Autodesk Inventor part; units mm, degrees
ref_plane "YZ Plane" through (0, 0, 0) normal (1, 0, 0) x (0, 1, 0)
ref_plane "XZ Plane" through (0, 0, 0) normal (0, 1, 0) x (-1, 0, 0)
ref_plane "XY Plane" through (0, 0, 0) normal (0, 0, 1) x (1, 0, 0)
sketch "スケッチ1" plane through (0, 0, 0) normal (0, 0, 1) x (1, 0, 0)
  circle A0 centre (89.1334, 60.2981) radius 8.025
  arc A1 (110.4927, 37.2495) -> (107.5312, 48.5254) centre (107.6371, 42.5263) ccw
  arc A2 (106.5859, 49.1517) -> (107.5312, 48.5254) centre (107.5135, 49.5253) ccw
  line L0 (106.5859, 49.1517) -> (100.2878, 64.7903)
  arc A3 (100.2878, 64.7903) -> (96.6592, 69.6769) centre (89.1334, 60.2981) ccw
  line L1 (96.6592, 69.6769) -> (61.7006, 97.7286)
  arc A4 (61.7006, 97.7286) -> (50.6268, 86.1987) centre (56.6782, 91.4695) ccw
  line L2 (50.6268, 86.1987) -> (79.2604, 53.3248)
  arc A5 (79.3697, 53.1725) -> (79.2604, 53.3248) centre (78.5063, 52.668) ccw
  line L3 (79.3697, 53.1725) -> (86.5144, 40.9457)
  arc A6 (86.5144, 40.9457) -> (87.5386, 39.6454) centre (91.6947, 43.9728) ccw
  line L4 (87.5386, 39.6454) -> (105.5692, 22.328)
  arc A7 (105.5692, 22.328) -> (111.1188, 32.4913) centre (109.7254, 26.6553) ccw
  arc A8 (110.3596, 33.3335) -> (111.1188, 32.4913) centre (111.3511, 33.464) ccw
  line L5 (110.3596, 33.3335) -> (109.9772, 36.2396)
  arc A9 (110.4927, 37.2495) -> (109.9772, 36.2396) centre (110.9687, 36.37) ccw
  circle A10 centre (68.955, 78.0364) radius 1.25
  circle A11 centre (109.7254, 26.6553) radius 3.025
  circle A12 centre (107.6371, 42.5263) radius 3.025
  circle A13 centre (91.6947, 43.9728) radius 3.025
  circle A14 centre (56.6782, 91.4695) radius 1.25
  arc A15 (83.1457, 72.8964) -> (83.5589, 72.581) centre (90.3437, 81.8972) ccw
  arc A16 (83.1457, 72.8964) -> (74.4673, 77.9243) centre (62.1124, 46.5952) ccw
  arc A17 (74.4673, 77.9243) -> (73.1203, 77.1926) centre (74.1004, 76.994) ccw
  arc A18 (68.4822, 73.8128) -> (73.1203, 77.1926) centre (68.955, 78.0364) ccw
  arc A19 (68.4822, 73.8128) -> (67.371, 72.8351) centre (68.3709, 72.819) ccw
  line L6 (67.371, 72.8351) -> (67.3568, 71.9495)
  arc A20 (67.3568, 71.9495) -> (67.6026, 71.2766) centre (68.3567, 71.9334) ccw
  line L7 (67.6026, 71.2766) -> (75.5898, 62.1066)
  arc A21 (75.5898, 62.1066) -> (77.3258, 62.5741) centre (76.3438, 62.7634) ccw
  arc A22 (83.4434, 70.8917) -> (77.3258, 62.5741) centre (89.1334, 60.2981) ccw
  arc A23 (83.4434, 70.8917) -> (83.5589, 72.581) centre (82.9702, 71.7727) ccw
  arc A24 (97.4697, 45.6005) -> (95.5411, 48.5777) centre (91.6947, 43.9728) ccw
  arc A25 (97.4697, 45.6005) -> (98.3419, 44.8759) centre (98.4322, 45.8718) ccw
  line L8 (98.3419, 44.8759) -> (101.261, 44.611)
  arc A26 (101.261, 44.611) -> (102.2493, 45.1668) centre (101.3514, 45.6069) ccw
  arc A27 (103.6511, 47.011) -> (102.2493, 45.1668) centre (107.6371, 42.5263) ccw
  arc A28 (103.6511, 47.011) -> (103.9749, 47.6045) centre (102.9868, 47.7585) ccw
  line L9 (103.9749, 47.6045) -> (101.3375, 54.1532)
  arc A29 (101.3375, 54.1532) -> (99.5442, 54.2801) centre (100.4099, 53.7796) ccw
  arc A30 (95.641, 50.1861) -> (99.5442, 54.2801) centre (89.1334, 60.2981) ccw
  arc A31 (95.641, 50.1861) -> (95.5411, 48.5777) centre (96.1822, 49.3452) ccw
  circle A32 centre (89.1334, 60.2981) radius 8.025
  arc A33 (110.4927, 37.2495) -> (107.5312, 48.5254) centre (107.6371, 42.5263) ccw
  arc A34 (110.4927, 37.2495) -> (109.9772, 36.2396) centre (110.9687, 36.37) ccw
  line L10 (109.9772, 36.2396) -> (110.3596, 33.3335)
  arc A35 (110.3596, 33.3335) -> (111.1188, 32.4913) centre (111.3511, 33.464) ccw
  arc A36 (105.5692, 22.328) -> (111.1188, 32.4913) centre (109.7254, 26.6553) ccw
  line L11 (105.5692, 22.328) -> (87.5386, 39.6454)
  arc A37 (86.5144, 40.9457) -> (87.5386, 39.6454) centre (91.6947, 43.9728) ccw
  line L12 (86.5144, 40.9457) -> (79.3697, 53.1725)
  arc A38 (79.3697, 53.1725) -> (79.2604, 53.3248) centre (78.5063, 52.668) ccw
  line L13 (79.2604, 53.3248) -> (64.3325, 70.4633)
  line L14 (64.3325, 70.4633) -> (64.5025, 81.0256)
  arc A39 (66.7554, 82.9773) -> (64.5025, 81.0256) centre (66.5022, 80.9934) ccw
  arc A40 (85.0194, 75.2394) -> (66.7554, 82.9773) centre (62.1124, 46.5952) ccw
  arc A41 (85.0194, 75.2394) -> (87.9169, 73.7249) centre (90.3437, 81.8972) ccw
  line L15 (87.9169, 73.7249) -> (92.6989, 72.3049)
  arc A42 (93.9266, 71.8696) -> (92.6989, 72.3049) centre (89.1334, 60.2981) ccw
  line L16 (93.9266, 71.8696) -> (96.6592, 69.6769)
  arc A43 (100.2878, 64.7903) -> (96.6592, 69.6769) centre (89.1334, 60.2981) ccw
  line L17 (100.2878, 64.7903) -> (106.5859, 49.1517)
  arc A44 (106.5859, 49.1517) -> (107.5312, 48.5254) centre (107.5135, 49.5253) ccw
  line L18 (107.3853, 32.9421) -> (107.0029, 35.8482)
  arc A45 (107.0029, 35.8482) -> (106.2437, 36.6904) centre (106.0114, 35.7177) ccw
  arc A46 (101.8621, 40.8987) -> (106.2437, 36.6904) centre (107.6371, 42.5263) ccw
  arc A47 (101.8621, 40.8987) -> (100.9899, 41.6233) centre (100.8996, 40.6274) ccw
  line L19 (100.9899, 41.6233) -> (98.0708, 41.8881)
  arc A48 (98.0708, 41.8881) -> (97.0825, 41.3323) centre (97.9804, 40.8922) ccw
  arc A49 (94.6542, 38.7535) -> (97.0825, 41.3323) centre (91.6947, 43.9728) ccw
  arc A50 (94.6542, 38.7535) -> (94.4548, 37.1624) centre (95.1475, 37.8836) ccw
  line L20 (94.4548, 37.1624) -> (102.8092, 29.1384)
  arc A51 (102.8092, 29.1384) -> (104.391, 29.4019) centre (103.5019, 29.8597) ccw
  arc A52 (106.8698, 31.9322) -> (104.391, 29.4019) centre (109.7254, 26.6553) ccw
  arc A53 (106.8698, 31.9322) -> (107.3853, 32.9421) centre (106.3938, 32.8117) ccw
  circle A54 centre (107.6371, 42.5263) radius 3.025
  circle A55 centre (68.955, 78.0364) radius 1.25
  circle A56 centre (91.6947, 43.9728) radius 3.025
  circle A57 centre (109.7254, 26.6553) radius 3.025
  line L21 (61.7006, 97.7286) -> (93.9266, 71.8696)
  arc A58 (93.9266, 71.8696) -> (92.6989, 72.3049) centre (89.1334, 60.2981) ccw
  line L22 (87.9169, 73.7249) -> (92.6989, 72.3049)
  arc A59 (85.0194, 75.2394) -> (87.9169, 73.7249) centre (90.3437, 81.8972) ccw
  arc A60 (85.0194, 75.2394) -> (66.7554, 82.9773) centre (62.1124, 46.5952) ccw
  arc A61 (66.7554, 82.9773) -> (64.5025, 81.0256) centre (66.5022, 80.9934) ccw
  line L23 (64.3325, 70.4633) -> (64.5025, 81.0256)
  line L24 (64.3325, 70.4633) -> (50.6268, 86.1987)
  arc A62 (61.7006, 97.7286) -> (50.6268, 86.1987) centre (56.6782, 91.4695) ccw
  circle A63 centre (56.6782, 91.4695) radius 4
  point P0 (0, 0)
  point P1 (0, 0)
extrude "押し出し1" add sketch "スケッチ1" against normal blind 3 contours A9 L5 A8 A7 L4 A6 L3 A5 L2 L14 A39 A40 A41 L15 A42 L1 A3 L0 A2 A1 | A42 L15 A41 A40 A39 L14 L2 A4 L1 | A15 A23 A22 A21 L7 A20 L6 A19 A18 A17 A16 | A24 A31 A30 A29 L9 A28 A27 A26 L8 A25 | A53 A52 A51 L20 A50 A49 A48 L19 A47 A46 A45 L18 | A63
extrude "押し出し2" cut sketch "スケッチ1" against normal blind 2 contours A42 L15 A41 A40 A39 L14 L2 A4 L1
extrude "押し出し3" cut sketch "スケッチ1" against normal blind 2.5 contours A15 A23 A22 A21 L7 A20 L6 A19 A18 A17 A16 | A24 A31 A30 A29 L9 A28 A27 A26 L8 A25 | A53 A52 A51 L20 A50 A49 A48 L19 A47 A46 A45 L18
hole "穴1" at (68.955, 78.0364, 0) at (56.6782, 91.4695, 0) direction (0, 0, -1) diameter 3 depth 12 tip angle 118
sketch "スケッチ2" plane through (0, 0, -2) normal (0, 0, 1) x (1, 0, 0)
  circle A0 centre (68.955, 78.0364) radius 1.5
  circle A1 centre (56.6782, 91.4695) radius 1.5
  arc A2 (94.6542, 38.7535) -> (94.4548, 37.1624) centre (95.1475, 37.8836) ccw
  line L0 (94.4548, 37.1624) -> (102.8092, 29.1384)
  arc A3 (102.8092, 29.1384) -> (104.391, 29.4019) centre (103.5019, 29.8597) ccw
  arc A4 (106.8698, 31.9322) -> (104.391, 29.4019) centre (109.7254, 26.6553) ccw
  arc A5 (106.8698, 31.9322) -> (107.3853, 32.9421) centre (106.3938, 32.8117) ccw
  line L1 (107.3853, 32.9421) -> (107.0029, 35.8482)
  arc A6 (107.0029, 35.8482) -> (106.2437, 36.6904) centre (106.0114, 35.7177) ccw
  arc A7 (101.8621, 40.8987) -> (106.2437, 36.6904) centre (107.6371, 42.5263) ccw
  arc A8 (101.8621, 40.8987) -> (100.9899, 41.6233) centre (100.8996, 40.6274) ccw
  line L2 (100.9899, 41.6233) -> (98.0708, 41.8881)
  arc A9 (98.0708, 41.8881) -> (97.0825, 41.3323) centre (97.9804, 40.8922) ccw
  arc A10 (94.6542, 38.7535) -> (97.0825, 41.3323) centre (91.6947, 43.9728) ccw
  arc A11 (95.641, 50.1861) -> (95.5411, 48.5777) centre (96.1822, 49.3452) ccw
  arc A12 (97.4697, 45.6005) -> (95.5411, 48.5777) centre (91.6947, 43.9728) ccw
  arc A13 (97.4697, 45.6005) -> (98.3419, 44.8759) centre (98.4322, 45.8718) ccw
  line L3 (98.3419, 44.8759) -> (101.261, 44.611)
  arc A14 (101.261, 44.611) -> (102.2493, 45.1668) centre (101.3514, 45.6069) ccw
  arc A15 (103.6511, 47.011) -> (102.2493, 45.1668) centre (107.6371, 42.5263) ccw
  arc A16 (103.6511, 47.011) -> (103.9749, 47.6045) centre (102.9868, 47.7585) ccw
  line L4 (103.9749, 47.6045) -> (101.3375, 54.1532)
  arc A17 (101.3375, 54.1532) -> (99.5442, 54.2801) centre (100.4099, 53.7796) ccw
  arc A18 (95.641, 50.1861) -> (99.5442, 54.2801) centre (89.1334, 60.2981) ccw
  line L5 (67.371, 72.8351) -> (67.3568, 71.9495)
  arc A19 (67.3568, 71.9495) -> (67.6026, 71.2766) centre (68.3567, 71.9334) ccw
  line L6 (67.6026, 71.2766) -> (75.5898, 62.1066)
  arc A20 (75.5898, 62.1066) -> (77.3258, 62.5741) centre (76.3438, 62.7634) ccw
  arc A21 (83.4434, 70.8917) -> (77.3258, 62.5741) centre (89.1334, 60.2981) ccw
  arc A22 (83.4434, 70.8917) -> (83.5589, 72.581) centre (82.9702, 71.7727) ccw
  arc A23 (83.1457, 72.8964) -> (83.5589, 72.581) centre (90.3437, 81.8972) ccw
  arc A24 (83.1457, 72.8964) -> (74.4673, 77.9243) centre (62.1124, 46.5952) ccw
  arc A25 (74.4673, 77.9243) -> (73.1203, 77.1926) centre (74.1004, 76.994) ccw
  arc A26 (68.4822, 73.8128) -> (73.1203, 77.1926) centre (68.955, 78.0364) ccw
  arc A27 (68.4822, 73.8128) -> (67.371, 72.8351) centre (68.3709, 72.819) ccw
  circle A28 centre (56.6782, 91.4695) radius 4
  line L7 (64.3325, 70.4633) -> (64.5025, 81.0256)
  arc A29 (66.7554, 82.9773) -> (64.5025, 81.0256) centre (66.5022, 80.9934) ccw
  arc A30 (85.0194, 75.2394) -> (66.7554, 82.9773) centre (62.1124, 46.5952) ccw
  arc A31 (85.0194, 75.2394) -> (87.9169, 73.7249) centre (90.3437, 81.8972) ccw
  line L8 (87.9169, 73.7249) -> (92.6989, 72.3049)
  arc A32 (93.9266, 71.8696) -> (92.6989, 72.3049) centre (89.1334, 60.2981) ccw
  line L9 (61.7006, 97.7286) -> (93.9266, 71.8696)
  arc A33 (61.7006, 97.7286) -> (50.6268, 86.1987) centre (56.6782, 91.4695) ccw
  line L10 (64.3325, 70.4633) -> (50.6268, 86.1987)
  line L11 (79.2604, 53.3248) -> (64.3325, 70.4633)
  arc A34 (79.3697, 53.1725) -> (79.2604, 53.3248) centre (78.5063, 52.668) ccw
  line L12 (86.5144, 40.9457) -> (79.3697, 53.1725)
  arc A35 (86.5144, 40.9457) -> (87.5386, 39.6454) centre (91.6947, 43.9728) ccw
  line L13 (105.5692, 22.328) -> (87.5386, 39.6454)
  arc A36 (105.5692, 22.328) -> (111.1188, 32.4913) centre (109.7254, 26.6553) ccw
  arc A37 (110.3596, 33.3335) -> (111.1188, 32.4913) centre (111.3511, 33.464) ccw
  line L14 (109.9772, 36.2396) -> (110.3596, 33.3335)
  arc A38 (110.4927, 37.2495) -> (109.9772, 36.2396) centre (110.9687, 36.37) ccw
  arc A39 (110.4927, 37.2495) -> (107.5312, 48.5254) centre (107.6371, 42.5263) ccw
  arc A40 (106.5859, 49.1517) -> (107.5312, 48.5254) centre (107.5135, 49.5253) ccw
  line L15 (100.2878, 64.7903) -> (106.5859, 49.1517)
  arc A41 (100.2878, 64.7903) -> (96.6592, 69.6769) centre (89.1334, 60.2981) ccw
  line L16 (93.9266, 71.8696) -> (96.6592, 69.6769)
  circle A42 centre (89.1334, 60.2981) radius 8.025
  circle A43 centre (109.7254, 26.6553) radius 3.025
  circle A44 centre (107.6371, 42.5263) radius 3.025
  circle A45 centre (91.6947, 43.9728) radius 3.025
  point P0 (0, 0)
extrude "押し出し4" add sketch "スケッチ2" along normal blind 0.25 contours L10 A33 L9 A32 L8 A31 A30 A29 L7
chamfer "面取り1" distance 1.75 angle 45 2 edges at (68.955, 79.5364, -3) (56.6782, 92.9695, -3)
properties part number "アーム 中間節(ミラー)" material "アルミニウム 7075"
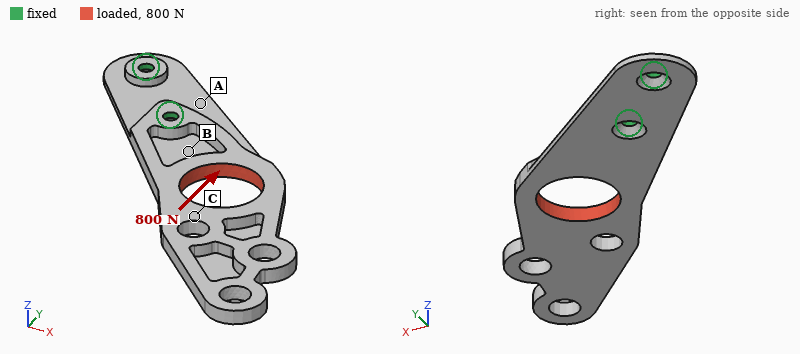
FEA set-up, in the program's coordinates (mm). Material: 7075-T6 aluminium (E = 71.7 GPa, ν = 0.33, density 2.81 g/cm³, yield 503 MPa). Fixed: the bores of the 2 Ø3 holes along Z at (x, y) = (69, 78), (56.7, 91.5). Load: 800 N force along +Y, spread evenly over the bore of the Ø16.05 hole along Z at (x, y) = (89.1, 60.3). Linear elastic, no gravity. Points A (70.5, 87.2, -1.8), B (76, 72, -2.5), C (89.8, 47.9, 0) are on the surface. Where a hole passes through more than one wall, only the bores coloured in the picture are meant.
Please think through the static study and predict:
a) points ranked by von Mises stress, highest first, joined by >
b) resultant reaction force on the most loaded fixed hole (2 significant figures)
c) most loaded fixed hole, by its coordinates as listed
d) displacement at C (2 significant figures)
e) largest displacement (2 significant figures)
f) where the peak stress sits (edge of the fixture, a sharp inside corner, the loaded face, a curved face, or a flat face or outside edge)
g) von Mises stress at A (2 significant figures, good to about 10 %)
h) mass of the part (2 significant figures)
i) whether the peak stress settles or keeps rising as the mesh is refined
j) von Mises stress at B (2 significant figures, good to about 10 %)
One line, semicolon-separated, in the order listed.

B > A > C; 1.2 kN; (69, 78); 0.36 mm; 0.69 mm; edge of the fixture; 110 MPa; 9.0 g; keeps rising; 160 MPa
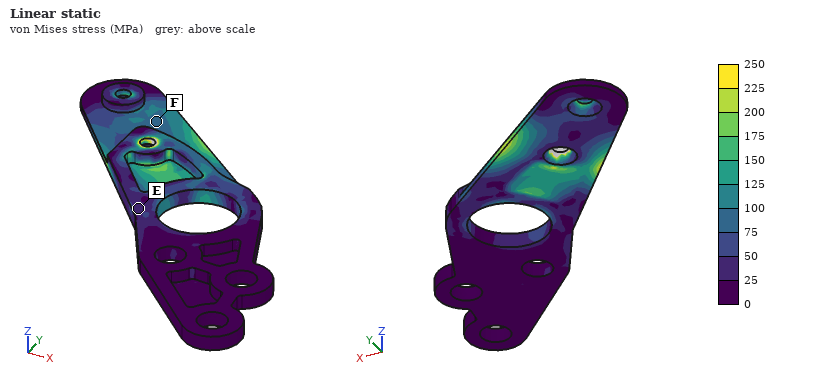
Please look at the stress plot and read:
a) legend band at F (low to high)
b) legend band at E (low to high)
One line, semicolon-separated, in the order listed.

75 to 100 MPa; 25 to 50 MPa
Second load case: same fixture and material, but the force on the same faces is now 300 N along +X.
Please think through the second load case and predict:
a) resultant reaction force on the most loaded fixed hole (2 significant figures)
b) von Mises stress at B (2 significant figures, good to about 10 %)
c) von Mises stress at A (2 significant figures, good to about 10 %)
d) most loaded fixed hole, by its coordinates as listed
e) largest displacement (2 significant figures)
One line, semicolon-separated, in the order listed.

470 N; 53 MPa; 32 MPa; (69, 78); 0.18 mm
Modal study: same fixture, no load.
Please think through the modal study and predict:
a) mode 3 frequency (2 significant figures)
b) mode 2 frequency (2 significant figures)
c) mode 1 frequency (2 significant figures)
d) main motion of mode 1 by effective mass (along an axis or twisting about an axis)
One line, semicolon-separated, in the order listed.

2200 Hz; 2000 Hz; 420 Hz; along Z
